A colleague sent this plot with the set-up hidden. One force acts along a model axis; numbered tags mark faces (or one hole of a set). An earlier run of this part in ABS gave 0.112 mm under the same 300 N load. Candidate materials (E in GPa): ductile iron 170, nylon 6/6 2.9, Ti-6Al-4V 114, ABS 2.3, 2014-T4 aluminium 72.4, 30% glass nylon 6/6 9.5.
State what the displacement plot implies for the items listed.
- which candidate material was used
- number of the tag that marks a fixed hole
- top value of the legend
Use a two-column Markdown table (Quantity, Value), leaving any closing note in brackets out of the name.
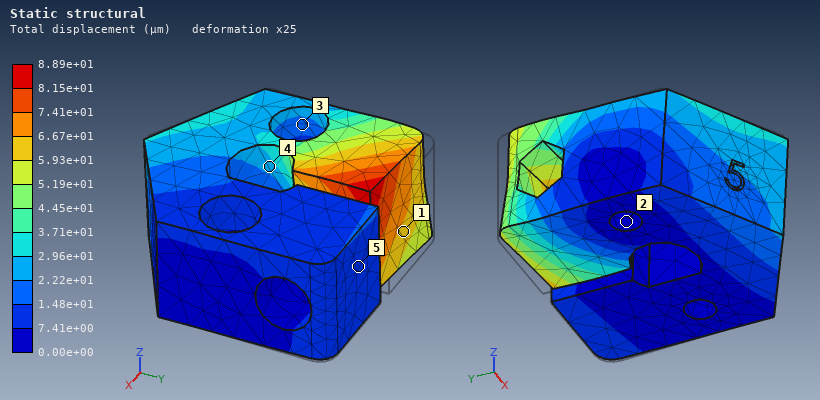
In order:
| Quantity | Value |
|---|---|
| which candidate material was used | nylon 6/6 |
| number of the tag that marks a fixed hole | 2 |
| top value of the legend | 8.89e+01 µm |
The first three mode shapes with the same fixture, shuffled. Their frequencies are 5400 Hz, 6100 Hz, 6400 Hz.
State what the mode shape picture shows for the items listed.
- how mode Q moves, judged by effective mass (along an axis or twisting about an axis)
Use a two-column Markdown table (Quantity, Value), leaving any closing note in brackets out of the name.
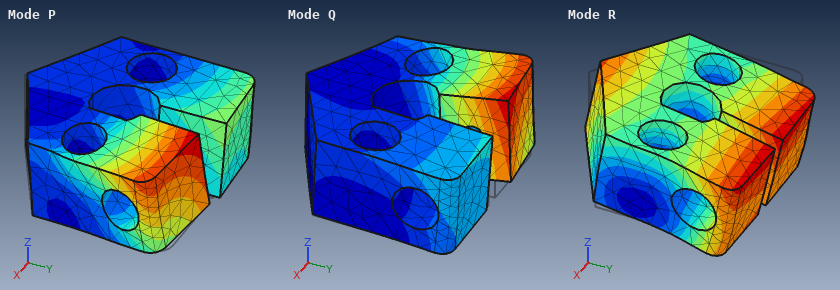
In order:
| Quantity | Value |
|---|---|
| how mode Q moves, judged by effective mass | along X |
